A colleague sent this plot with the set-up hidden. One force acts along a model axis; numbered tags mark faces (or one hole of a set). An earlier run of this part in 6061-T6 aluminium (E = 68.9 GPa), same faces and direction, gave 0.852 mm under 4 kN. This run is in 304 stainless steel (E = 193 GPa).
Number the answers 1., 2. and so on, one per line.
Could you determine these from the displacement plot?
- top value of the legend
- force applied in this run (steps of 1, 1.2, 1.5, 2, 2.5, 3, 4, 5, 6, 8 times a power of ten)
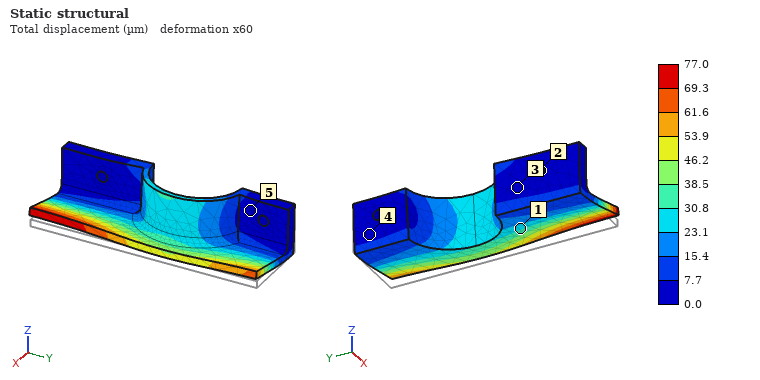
1. 77.0 µm
2. 1 kN
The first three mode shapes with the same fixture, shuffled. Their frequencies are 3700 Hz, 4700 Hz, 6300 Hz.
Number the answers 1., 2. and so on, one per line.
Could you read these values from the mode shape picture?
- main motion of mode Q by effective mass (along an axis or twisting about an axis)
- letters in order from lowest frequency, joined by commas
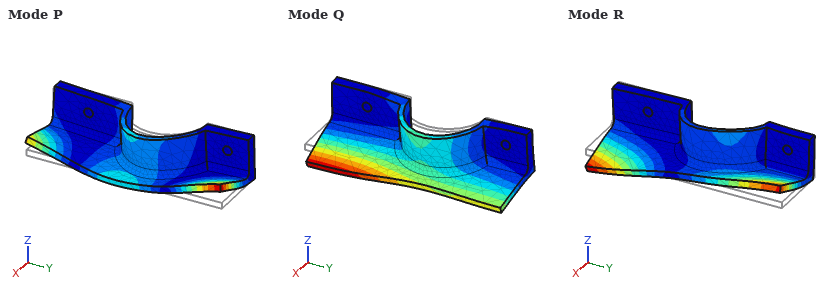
1. along Z
2. Q, R, P
